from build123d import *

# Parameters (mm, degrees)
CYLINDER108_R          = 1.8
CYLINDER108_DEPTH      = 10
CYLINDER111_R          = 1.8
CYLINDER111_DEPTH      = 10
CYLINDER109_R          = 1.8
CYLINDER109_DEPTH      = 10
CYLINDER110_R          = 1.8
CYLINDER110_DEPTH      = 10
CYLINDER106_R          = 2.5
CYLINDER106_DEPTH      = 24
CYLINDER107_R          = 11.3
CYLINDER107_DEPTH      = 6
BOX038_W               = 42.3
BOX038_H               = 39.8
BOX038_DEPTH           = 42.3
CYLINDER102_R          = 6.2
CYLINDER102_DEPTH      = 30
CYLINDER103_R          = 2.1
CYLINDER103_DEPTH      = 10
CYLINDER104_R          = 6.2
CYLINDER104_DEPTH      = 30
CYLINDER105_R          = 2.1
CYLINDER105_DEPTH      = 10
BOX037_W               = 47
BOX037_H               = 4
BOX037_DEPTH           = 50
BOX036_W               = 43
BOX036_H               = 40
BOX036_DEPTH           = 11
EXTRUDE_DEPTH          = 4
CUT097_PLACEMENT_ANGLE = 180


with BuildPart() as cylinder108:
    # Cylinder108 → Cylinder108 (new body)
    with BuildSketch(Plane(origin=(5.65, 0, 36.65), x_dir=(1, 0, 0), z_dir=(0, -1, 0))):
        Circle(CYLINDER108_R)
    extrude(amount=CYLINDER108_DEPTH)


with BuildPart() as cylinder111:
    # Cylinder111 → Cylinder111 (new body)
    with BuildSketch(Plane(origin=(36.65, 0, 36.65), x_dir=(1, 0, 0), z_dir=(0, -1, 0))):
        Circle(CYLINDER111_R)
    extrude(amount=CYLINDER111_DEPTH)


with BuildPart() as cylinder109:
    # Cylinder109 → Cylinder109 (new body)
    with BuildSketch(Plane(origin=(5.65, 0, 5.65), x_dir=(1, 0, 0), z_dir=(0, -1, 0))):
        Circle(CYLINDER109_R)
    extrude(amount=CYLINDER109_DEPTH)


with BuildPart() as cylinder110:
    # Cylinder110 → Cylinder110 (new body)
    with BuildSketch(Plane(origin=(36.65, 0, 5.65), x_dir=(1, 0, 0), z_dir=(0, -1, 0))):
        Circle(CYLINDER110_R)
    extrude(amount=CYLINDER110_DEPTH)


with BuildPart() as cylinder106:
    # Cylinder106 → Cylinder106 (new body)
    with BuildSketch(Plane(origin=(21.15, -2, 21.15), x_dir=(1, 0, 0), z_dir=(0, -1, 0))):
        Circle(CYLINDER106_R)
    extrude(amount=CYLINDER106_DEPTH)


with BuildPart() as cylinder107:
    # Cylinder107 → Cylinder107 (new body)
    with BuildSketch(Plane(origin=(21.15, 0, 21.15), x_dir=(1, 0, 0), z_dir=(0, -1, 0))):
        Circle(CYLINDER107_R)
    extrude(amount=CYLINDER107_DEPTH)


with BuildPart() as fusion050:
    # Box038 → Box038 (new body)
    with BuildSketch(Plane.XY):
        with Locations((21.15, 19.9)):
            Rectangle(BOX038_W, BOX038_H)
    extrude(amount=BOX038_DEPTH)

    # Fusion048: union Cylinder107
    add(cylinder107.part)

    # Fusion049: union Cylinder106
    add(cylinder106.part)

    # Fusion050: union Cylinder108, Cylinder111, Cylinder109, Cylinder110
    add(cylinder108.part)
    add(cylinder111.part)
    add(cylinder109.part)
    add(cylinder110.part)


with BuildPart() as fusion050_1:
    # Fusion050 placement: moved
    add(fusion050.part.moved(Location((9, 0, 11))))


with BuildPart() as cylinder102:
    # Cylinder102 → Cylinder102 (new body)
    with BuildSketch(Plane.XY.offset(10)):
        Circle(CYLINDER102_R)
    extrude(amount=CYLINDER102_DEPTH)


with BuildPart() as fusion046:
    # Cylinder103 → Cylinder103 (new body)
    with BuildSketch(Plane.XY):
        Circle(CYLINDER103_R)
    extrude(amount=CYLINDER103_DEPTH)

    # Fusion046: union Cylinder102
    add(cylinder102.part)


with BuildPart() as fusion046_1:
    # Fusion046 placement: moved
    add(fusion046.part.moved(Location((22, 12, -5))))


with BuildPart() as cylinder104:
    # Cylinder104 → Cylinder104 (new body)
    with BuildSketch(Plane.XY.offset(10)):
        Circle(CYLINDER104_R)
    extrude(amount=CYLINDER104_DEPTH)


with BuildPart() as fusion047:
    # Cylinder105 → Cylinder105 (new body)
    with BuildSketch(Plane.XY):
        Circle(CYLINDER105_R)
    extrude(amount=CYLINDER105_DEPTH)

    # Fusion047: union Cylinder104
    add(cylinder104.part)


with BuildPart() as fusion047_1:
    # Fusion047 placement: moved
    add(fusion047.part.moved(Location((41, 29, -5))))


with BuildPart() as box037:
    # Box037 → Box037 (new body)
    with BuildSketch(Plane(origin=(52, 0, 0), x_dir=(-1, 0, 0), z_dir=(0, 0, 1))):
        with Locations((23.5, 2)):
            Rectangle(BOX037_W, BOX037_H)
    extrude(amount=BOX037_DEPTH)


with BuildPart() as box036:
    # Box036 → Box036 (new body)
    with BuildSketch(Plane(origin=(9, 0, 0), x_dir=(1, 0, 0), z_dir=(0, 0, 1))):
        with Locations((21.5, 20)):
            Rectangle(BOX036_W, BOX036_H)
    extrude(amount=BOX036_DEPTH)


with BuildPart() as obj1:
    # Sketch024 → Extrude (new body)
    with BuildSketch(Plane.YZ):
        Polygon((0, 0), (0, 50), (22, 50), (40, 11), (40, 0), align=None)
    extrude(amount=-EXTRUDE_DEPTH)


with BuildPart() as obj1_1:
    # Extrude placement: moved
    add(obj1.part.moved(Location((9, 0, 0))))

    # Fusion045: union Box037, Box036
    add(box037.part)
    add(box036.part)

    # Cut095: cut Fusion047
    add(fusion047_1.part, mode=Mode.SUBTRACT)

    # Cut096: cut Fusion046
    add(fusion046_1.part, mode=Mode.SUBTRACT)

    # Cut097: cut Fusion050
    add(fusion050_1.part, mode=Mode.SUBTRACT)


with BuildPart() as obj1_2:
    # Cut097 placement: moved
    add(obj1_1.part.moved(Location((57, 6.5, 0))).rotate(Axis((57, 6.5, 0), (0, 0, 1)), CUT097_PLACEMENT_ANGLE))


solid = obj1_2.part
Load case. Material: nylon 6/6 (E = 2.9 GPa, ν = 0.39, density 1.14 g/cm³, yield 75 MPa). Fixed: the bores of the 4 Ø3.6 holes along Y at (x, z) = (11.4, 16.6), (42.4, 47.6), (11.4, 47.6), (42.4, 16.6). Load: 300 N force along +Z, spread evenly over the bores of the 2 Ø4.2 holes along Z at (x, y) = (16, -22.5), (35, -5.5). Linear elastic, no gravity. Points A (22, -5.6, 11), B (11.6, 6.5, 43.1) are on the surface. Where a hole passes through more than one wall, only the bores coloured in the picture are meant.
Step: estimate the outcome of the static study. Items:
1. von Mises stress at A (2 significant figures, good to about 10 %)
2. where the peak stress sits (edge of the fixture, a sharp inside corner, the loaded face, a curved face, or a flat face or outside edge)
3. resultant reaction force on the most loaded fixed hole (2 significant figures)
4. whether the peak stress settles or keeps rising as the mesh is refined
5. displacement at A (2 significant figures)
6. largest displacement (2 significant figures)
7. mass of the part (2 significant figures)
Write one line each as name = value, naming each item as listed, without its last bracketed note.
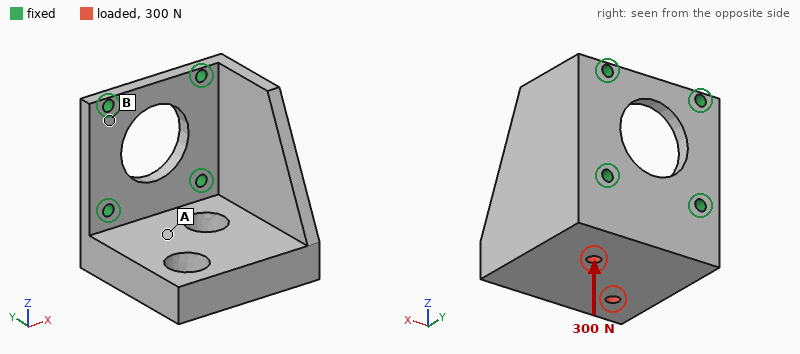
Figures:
von Mises stress at A = 5.7 MPa
where the peak stress sits = edge of the fixture
resultant reaction force on the most loaded fixed hole = 220 N
whether the peak stress settles or keeps rising as the mesh is refined = keeps rising
displacement at A = 0.23 mm
largest displacement = 0.83 mm
mass of the part = 36 g
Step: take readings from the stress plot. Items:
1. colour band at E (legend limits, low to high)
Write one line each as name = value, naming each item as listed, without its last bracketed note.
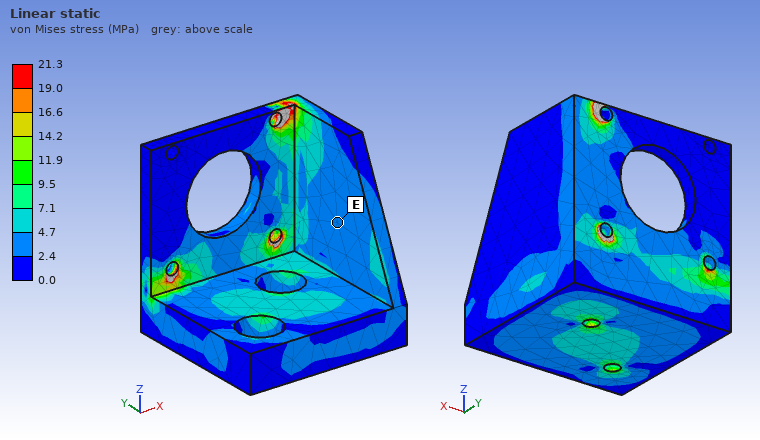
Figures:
colour band at E = 2.4 to 4.7 MPa
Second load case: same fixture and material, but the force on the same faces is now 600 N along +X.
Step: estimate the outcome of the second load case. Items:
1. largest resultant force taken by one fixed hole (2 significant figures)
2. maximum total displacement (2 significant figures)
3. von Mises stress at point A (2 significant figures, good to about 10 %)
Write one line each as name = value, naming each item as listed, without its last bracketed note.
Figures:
largest resultant force taken by one fixed hole = 560 N
maximum total displacement = 0.45 mm
von Mises stress at point A = 4.9 MPa
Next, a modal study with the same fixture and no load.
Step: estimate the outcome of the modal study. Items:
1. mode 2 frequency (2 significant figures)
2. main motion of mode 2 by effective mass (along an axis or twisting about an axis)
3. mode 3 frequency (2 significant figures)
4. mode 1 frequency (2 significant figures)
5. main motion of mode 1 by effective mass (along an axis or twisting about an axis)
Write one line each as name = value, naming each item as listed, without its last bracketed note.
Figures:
mode 2 frequency = 1200 Hz
main motion of mode 2 by effective mass = along X
mode 3 frequency = 1900 Hz
mode 1 frequency = 890 Hz
main motion of mode 1 by effective mass = along Z
